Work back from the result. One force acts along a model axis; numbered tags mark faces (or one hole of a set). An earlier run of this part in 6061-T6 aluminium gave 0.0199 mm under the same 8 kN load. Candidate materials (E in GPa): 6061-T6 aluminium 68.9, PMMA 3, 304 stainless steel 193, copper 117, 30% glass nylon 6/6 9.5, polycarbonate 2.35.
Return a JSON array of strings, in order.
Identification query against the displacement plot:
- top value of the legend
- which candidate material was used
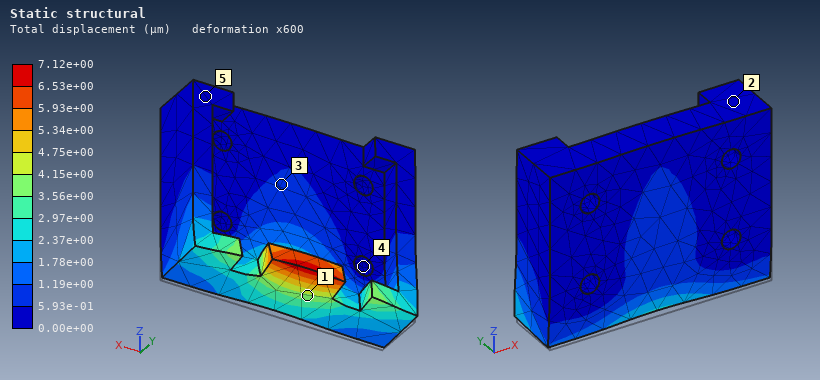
["7.12e+00 µm", "304 stainless steel"]
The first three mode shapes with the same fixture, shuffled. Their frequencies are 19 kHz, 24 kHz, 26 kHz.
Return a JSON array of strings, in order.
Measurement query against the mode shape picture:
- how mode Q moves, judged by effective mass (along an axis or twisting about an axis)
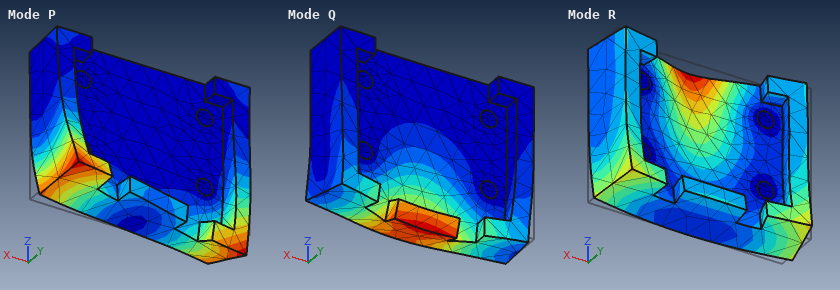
["along Y"]
